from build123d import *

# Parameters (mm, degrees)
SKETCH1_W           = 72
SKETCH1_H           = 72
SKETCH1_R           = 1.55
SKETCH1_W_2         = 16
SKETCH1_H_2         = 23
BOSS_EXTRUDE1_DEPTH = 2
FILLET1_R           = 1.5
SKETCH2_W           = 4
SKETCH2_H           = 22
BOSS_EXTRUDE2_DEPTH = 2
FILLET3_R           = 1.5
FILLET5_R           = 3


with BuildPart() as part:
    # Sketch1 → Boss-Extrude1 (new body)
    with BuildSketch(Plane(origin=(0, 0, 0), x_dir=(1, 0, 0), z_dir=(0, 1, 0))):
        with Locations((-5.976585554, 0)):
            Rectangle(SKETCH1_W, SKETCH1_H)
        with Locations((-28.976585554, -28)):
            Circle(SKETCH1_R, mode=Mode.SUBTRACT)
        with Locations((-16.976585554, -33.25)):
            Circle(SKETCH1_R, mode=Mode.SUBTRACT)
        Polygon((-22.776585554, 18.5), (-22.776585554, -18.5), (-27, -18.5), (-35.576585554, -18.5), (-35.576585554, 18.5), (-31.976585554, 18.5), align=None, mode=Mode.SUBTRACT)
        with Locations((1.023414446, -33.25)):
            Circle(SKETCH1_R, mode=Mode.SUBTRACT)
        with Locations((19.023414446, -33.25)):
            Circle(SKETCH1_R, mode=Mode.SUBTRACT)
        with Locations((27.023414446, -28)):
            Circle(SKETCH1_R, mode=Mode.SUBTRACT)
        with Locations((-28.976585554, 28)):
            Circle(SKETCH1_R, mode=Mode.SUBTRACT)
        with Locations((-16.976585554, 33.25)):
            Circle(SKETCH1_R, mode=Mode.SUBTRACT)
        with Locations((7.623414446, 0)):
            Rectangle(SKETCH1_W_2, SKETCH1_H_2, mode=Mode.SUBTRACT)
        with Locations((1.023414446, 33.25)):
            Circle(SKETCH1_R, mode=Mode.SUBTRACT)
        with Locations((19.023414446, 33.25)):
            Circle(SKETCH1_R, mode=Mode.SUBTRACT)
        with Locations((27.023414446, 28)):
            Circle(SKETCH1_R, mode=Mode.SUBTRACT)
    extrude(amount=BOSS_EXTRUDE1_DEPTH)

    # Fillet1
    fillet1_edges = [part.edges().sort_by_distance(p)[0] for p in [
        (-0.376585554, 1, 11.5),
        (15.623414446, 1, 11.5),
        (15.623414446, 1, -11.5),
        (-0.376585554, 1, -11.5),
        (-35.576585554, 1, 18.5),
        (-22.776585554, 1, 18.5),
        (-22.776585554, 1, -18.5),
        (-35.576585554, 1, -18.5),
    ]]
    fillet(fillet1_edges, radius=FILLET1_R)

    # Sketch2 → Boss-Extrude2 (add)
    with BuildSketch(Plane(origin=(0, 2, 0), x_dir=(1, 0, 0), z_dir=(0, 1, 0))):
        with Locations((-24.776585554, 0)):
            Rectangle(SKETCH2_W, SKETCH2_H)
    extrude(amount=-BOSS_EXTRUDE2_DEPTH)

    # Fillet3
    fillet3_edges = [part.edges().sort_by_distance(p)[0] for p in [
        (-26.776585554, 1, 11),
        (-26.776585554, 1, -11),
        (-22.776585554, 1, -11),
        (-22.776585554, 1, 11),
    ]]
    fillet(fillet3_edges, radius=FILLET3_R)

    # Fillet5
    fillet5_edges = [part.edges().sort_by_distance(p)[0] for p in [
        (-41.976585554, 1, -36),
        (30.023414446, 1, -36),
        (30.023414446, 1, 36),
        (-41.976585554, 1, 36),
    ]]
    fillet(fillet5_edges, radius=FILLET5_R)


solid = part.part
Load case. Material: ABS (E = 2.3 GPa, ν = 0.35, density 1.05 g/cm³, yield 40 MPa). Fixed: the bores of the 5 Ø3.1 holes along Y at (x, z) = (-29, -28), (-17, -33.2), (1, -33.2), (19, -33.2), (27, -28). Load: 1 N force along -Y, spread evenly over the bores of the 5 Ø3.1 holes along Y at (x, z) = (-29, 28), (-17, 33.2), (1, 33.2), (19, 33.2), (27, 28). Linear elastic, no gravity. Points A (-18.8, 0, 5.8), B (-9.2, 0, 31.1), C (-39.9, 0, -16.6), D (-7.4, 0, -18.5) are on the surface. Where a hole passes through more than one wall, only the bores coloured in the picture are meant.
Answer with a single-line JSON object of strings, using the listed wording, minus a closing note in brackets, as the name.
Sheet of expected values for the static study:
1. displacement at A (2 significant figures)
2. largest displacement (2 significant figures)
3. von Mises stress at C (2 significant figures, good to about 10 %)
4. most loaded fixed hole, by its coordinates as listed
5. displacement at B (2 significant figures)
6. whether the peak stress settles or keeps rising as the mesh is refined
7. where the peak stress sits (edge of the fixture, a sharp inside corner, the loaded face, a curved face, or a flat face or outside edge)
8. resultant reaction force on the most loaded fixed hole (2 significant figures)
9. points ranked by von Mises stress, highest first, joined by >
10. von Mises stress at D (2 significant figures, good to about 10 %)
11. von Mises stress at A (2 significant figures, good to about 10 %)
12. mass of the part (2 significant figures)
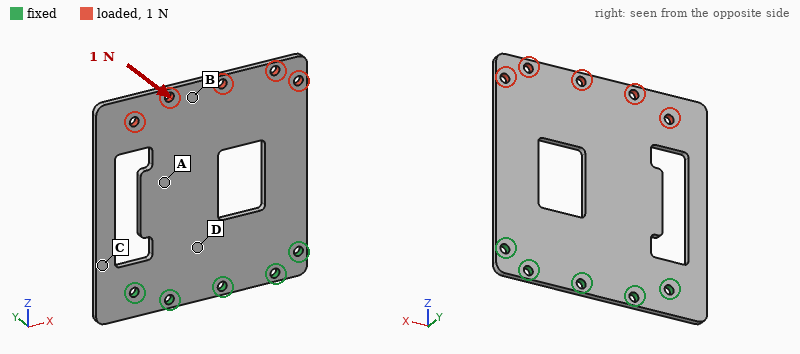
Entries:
{"displacement at A": "0.35 mm", "largest displacement": "1.0 mm", "von Mises stress at C": "1.5 MPa", "most loaded fixed hole, by its coordinates as listed": "(27, -28)", "displacement at B": "0.90 mm", "whether the peak stress settles or keeps rising as the mesh is refined": "keeps rising", "where the peak stress sits": "edge of the fixture", "resultant reaction force on the most loaded fixed hole": "0.97 N", "points ranked by von Mises stress, highest first, joined by >": "C > D > A > B", "von Mises stress at D": "1.1 MPa", "von Mises stress at A": "0.73 MPa", "mass of the part": "9.1 g"}
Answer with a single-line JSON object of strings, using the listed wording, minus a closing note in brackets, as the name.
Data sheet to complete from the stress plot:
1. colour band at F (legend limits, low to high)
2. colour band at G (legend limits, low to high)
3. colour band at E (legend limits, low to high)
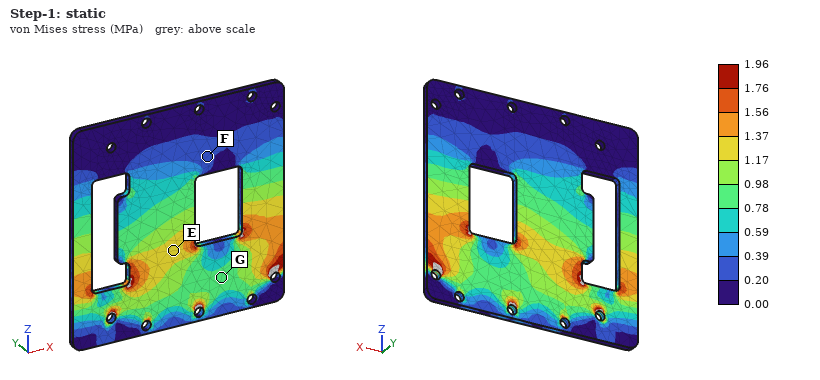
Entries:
{"colour band at F": "0.20 to 0.39 MPa", "colour band at G": "0.78 to 0.98 MPa", "colour band at E": "1.17 to 1.37 MPa"}
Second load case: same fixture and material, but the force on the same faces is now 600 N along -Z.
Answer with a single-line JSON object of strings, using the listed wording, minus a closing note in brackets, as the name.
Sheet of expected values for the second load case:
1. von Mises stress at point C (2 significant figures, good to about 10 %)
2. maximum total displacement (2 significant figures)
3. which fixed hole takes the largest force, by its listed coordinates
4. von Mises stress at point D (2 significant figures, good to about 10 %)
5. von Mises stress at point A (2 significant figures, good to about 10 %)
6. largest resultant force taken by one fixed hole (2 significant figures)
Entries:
{"von Mises stress at point C": "3.3 MPa", "maximum total displacement": "0.23 mm", "which fixed hole takes the largest force, by its listed coordinates": "(27, -28)", "von Mises stress at point D": "4.6 MPa", "von Mises stress at point A": "5.8 MPa", "largest resultant force taken by one fixed hole": "150 N"}
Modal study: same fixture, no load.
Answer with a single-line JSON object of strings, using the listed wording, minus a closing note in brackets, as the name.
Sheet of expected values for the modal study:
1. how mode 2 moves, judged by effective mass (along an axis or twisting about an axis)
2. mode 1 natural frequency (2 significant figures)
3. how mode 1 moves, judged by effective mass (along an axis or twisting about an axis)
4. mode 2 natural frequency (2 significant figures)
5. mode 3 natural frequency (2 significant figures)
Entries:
{"how mode 2 moves, judged by effective mass": "twisting about Z", "mode 1 natural frequency": "100 Hz", "how mode 1 moves, judged by effective mass": "along Y", "mode 2 natural frequency": "240 Hz", "mode 3 natural frequency": "630 Hz"}
